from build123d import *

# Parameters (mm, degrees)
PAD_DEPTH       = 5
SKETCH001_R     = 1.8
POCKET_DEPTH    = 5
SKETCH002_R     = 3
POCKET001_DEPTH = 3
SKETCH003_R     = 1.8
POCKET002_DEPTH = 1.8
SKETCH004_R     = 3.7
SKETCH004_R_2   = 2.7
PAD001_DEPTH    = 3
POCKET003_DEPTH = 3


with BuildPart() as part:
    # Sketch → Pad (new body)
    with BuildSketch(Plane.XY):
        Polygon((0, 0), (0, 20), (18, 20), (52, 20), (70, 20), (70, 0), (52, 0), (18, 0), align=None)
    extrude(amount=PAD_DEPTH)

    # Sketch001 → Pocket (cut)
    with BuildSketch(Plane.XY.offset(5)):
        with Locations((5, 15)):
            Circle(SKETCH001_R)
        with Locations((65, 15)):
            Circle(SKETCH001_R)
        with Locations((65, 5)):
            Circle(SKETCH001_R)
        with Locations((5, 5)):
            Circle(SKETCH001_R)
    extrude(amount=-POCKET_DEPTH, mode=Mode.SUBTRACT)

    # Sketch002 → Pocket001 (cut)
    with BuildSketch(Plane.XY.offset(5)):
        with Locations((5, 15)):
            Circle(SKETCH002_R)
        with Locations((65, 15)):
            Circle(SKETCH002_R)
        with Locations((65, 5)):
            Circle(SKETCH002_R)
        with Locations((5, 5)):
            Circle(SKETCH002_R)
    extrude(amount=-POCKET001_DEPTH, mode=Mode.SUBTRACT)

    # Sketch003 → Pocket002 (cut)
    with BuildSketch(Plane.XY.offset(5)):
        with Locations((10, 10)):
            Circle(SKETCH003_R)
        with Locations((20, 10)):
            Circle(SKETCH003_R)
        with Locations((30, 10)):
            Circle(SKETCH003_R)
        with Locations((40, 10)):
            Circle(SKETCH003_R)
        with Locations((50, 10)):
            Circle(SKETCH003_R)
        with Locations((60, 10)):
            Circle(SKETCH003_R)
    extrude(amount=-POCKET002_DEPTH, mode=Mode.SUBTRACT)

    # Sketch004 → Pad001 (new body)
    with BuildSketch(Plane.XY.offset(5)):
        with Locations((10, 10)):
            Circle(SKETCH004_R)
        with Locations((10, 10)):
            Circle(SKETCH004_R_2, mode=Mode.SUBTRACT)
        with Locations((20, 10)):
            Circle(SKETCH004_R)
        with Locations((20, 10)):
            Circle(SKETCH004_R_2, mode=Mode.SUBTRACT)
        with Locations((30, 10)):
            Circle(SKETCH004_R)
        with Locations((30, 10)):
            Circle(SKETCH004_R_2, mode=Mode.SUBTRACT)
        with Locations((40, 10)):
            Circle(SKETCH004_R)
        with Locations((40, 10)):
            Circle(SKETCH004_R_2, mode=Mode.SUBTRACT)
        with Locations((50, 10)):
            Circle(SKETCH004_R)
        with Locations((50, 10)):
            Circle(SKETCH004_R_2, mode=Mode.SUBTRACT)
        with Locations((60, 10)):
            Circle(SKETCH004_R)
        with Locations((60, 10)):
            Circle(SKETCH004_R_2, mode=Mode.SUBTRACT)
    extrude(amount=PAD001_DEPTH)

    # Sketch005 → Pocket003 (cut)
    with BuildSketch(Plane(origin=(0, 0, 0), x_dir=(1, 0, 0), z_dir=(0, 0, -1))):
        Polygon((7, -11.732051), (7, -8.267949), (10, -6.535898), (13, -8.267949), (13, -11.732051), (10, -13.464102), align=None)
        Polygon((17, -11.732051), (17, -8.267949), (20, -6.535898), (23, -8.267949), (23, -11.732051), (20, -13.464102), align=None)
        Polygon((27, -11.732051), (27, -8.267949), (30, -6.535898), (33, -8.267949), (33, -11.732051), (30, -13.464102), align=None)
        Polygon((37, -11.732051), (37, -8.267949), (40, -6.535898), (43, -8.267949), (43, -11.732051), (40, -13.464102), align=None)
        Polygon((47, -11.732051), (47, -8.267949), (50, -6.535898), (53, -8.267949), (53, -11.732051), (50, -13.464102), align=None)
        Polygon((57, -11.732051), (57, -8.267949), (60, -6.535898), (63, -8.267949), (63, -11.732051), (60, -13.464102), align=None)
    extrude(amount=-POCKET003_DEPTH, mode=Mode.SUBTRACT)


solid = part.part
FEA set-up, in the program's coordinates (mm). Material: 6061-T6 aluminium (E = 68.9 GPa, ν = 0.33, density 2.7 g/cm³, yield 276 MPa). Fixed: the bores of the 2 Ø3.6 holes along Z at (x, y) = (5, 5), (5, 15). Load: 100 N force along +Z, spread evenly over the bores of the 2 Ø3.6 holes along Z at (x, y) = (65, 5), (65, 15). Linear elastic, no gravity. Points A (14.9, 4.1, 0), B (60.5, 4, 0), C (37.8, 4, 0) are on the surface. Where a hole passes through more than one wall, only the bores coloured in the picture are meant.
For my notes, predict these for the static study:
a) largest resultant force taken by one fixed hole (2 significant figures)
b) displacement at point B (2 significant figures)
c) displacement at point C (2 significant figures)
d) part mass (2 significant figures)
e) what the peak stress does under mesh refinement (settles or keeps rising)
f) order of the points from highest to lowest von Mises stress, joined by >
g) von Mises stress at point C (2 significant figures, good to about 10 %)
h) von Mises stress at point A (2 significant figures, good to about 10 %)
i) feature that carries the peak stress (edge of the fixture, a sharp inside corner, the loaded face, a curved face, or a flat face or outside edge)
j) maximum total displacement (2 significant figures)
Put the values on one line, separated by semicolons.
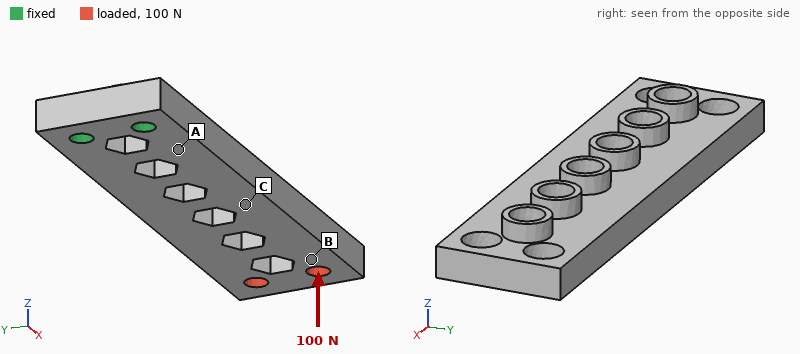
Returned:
55 N; 0.70 mm; 0.32 mm; 17 g; keeps rising; A > C > B; 41 MPa; 73 MPa; edge of the fixture; 0.87 mm
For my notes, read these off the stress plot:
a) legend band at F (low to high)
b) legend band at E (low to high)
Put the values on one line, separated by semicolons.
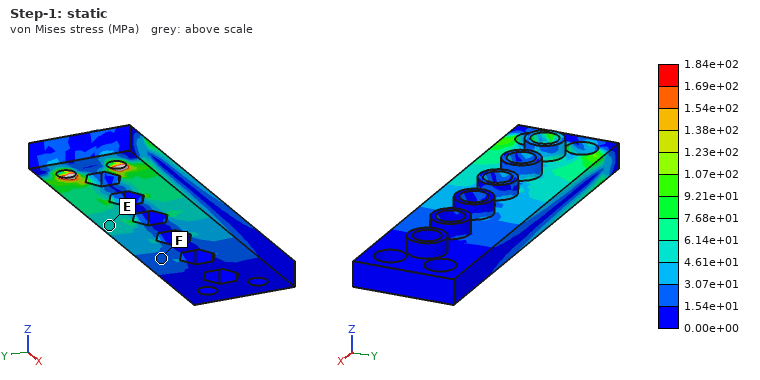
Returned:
1.54e+01 to 3.07e+01 MPa; 4.61e+01 to 6.14e+01 MPa
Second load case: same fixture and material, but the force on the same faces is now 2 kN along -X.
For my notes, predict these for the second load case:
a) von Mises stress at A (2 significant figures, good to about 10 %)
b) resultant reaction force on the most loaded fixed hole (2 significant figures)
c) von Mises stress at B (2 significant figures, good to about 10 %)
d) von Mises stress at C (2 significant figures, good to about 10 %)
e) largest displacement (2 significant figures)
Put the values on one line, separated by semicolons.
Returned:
75 MPa; 1.0 kN; 69 MPa; 74 MPa; 0.53 mm
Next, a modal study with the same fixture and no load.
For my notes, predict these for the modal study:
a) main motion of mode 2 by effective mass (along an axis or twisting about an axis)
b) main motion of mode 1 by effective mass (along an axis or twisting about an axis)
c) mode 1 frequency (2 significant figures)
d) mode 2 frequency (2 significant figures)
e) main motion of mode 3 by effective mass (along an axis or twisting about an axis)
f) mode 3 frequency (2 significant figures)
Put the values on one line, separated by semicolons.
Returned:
along Y; along Z; 810 Hz; 3000 Hz; twisting about X; 5000 Hz
